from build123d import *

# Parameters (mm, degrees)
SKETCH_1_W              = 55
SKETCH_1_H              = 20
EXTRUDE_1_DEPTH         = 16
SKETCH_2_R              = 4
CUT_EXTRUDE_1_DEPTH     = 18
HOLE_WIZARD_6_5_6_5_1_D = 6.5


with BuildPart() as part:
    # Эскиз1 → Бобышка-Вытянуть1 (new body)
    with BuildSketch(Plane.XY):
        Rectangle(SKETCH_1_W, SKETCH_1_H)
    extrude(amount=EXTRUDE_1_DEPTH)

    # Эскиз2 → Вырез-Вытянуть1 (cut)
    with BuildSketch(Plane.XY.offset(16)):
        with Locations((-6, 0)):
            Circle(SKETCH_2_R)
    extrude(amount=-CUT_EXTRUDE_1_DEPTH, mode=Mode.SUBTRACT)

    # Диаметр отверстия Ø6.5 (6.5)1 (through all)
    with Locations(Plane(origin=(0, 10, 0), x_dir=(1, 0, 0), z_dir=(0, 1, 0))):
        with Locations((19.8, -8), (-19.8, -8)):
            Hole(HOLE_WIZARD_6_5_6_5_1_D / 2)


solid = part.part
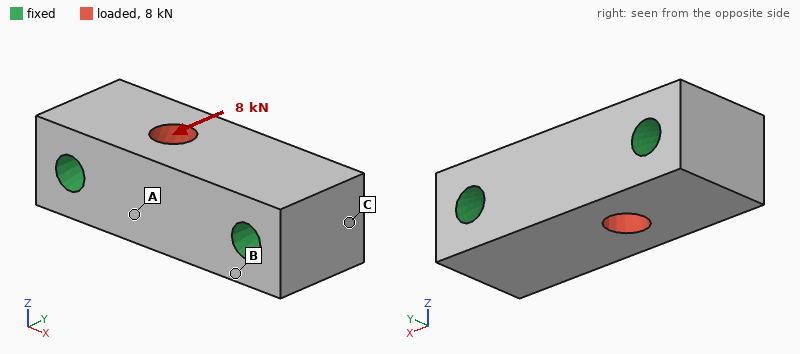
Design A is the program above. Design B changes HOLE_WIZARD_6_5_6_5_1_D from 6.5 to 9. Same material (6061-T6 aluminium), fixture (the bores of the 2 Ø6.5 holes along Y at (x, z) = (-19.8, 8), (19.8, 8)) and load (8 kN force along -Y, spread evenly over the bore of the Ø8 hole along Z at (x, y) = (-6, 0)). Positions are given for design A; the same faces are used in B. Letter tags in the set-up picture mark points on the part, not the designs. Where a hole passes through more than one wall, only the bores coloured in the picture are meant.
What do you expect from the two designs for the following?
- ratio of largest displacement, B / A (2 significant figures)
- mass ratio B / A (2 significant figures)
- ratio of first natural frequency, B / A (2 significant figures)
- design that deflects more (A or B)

0.88
0.92
1.2
A
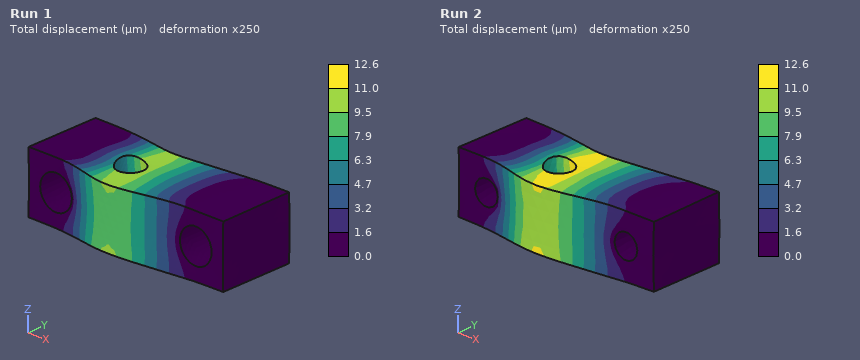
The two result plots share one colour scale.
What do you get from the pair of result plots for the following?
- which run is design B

Run 1
